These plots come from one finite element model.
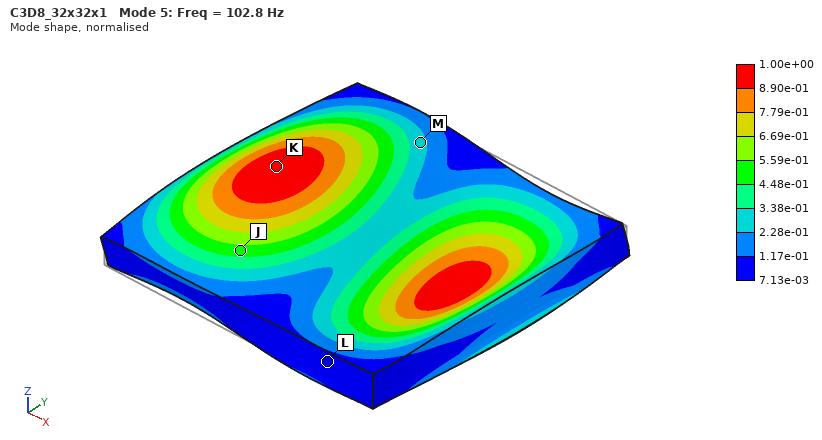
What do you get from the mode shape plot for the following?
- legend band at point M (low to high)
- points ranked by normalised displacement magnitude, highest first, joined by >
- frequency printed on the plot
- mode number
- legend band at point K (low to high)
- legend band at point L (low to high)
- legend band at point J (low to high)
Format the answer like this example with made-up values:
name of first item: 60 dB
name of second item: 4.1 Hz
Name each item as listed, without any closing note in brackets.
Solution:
legend band at point M: 2.28e-01 to 3.38e-01
points ranked by normalised displacement magnitude, highest first, joined by >: K > J > M > L
frequency printed on the plot: 102.8 Hz
mode number: 5
legend band at point K: 8.90e-01 to 1.00e+00
legend band at point L: 7.13e-03 to 1.17e-01
legend band at point J: 4.48e-01 to 5.59e-01
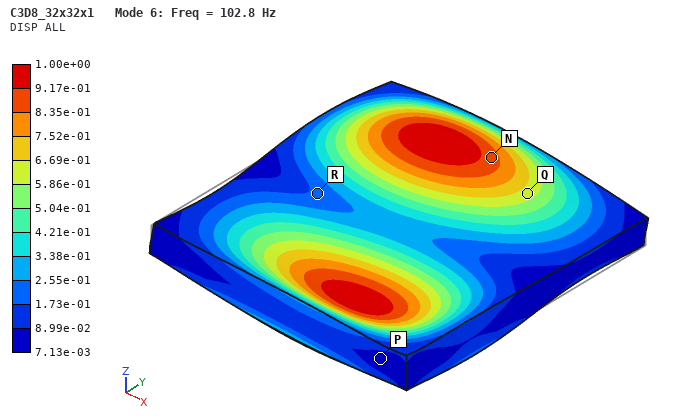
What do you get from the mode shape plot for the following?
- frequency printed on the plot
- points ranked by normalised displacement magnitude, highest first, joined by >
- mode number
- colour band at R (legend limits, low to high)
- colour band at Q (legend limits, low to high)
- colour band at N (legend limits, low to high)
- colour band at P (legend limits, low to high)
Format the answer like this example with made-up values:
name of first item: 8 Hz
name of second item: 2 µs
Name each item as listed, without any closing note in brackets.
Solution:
frequency printed on the plot: 102.8 Hz
points ranked by normalised displacement magnitude, highest first, joined by >: N > Q > R > P
mode number: 6
colour band at R: 1.73e-01 to 2.55e-01
colour band at Q: 5.86e-01 to 6.69e-01
colour band at N: 8.35e-01 to 9.17e-01
colour band at P: 7.13e-03 to 8.99e-02
